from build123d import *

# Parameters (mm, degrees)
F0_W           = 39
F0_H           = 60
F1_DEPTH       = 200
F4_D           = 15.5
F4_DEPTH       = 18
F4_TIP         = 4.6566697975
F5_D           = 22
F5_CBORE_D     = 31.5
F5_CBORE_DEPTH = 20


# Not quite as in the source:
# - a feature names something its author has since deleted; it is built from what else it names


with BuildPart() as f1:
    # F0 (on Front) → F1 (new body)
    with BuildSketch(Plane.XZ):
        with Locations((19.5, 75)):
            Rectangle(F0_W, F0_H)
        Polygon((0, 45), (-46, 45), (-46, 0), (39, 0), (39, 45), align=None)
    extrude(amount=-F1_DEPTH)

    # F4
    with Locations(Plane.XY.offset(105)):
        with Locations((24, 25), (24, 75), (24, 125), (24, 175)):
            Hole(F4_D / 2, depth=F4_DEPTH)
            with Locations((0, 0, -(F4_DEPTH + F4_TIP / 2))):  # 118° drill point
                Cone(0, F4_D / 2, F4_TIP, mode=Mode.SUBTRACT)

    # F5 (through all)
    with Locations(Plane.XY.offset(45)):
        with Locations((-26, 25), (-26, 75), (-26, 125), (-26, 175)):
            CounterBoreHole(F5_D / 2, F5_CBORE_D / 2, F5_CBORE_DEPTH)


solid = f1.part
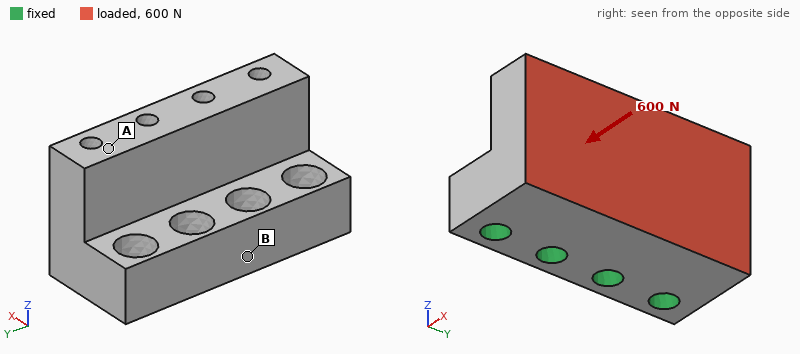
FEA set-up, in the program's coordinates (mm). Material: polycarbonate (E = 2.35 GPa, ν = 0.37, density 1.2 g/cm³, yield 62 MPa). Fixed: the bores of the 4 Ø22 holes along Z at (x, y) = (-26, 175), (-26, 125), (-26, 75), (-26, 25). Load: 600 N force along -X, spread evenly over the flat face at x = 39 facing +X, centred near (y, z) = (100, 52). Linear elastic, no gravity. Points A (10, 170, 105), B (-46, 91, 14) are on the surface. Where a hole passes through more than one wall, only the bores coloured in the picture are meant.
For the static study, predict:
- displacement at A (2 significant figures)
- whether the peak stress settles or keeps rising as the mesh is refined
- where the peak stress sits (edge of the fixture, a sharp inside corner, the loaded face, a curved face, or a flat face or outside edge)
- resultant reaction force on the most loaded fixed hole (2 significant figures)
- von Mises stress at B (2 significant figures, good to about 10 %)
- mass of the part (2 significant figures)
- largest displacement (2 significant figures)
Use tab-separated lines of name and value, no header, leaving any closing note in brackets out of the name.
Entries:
displacement at A	50 µm
whether the peak stress settles or keeps rising as the mesh is refined	keeps rising
where the peak stress sits	edge of the fixture
resultant reaction force on the most loaded fixed hole	160 N
von Mises stress at B	0.22 MPa
mass of the part	1.3 kg
largest displacement	57 µm
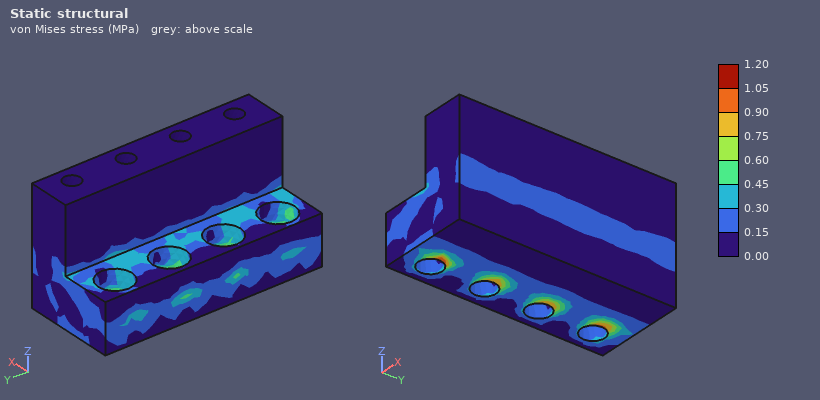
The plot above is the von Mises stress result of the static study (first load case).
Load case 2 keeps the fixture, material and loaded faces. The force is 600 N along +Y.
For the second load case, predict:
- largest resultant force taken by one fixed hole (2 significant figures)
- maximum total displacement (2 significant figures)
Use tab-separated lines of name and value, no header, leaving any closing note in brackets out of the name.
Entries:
largest resultant force taken by one fixed hole	280 N
maximum total displacement	14 µm
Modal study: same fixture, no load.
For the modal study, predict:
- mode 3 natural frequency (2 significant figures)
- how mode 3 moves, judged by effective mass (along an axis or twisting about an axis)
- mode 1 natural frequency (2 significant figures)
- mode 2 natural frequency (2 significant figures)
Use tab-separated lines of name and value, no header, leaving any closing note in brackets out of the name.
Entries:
mode 3 natural frequency	1500 Hz
how mode 3 moves, judged by effective mass	along Y
mode 1 natural frequency	580 Hz
mode 2 natural frequency	920 Hz
